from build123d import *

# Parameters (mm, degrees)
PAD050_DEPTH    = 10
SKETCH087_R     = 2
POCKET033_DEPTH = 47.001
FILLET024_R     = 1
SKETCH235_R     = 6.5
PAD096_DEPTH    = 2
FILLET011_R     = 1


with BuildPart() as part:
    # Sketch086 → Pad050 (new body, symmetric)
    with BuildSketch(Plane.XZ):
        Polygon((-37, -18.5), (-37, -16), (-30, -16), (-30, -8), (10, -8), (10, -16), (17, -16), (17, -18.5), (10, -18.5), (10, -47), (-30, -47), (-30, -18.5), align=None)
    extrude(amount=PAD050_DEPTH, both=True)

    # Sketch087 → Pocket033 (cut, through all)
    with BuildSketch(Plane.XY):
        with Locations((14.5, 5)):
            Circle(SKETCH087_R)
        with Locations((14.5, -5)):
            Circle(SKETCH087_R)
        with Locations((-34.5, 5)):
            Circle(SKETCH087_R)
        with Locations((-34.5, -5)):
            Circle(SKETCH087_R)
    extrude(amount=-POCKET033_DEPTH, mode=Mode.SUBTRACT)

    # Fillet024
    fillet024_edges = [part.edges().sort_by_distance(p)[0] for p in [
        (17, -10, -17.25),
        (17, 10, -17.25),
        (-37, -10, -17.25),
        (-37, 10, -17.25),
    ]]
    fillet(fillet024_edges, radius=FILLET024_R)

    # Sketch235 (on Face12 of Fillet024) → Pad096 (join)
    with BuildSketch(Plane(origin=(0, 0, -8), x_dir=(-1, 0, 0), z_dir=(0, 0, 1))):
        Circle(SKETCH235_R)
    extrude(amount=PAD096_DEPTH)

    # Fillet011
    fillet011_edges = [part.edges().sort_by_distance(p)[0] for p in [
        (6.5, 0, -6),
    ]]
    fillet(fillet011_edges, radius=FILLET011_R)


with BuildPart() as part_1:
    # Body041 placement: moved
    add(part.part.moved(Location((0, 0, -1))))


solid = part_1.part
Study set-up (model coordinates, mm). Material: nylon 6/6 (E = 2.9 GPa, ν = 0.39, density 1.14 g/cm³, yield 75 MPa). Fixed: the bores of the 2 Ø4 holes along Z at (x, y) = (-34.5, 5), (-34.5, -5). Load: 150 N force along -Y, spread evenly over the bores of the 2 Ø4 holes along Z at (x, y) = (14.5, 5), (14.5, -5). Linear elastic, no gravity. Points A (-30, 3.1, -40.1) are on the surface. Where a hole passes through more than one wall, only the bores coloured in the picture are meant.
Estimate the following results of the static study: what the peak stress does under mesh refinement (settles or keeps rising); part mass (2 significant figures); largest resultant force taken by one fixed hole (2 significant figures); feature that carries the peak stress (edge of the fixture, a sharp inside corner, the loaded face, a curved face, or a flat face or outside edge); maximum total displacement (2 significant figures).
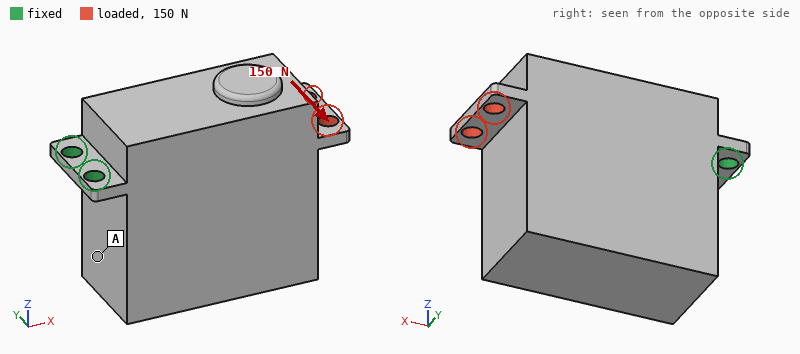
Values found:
keeps rising
37 g
590 N
edge of the fixture
0.70 mm
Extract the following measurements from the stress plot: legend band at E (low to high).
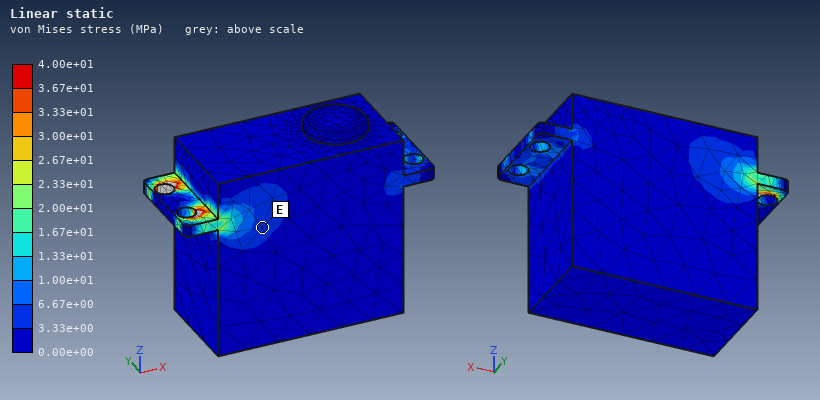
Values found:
3.33e+00 to 6.67e+00 MPa
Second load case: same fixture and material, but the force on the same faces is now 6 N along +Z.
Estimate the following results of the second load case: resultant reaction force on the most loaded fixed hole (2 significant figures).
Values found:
3.0 N
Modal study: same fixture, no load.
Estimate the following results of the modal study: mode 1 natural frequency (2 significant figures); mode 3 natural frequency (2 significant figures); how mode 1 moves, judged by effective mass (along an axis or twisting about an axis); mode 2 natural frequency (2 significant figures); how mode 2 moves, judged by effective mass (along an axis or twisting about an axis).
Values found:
130 Hz
1100 Hz
along Z
590 Hz
along Y
